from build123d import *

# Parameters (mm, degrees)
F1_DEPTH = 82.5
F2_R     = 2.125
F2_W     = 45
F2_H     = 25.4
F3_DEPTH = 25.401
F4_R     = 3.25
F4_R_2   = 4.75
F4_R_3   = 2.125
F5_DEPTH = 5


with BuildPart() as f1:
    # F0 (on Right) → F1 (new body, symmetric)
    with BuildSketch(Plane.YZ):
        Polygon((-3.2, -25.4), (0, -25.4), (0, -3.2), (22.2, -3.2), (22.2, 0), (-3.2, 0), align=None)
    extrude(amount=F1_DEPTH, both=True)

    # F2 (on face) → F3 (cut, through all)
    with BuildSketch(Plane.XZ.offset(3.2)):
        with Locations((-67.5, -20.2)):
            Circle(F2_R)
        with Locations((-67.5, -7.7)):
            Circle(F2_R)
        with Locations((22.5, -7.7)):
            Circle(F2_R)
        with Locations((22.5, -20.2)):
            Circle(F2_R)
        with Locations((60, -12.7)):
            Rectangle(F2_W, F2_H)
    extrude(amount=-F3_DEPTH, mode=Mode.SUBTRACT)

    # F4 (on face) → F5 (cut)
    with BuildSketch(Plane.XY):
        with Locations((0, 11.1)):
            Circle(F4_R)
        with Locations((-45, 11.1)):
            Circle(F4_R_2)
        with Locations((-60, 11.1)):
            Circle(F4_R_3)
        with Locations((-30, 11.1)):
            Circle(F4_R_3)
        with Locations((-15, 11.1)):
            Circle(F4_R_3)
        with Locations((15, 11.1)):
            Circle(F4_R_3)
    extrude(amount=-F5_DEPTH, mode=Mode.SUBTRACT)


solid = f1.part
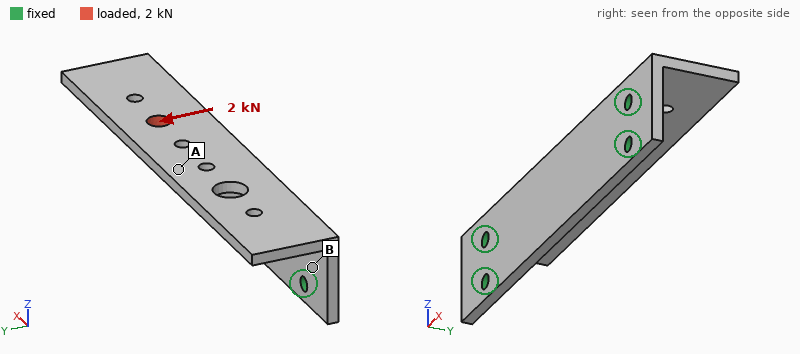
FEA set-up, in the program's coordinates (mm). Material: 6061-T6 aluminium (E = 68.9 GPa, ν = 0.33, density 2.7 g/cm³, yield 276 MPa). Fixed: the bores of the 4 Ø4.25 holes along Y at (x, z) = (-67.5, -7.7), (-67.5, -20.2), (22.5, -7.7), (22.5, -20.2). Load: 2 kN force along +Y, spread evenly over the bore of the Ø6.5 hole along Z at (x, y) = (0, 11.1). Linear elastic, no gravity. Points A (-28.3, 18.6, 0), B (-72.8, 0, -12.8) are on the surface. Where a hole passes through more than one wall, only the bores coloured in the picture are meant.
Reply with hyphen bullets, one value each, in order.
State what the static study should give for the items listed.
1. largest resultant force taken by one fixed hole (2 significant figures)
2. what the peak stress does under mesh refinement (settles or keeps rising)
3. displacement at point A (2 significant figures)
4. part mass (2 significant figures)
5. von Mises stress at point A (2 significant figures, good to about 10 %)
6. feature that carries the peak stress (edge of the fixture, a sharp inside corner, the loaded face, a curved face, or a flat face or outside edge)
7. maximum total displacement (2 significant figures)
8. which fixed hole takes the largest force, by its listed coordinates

- 2.1 kN
- keeps rising
- 0.095 mm
- 47 g
- 32 MPa
- edge of the fixture
- 0.13 mm
- (22.5, -7.7)
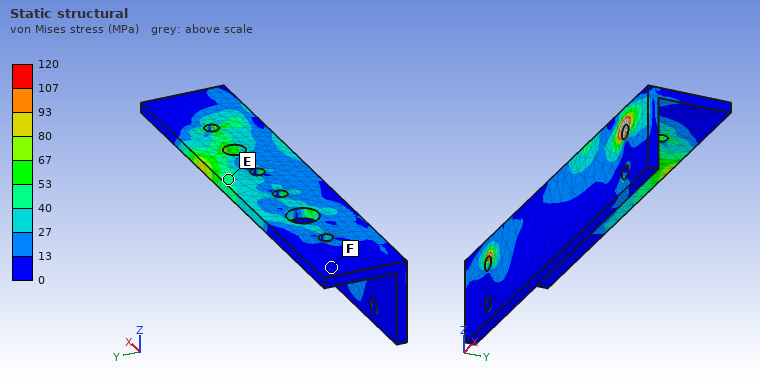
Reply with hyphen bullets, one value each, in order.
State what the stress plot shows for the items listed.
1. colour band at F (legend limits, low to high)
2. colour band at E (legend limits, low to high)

- 0 to 13 MPa
- 40 to 53 MPa
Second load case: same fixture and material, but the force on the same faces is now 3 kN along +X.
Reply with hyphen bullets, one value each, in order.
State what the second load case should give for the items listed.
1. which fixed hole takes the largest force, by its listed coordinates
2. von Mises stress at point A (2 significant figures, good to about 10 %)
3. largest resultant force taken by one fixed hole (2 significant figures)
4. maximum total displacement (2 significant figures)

- (22.5, -7.7)
- 24 MPa
- 1.4 kN
- 46 µm
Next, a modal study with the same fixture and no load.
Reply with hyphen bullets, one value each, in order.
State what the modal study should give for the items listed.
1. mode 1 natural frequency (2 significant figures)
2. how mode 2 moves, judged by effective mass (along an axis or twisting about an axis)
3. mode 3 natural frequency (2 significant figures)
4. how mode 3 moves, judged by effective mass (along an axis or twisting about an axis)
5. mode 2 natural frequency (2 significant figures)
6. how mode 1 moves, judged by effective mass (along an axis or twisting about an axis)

- 2500 Hz
- twisting about Y
- 4100 Hz
- along Y
- 3700 Hz
- along Z
